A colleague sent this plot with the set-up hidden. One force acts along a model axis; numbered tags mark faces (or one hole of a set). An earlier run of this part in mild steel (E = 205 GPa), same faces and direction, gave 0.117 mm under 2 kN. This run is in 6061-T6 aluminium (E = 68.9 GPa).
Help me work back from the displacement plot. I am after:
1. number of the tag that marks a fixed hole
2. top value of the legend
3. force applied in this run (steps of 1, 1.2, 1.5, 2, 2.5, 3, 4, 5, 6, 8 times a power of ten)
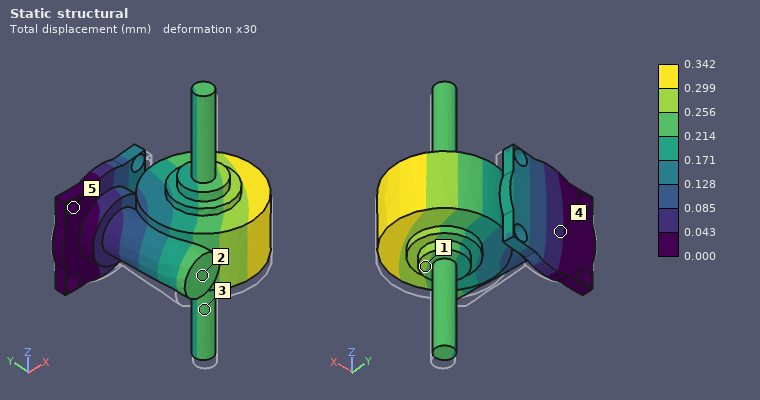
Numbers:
5
0.342 mm
2 kN
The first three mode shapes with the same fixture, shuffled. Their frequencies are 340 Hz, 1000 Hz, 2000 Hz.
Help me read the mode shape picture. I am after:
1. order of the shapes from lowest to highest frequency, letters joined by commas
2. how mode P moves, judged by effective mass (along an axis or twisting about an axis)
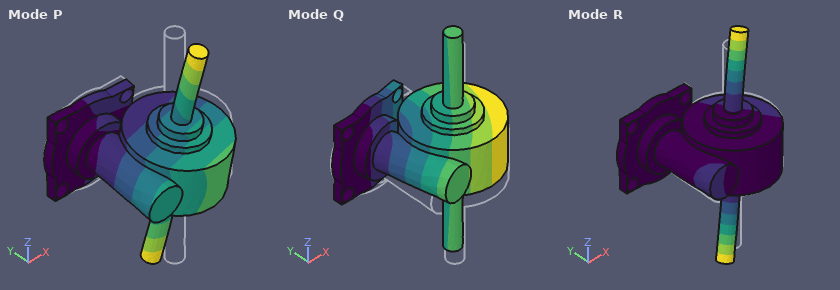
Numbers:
Q, P, R
along Z
